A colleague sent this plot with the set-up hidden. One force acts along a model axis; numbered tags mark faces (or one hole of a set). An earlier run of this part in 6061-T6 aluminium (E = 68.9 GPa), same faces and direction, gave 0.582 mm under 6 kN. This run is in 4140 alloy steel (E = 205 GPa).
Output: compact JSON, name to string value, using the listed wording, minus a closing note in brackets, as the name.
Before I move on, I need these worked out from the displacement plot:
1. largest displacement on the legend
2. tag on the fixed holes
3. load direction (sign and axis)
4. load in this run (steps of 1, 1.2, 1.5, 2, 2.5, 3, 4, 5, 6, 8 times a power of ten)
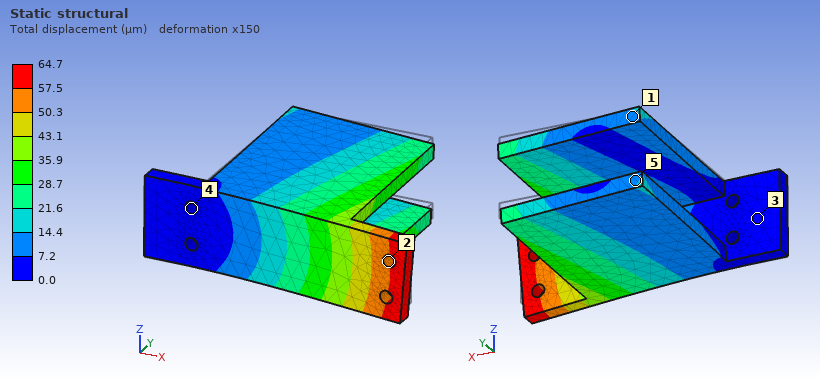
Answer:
{"largest displacement on the legend": "64.7 µm", "tag on the fixed holes": "4", "load direction": "-Z", "load in this run": "2 kN"}
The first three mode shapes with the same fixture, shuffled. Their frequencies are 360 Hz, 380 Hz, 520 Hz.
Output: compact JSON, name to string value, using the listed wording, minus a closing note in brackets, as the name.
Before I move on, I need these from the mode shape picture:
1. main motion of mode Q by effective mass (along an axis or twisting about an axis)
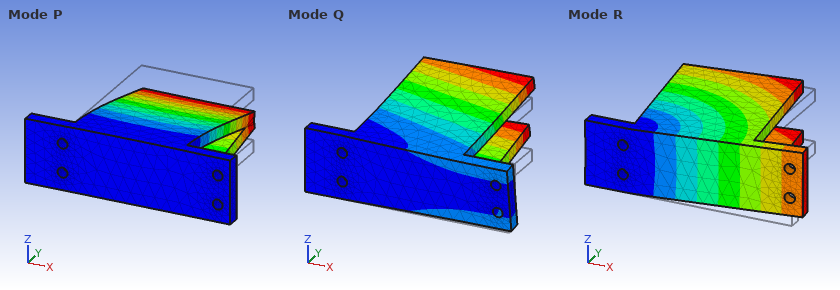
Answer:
{"main motion of mode Q by effective mass": "along Z"}
